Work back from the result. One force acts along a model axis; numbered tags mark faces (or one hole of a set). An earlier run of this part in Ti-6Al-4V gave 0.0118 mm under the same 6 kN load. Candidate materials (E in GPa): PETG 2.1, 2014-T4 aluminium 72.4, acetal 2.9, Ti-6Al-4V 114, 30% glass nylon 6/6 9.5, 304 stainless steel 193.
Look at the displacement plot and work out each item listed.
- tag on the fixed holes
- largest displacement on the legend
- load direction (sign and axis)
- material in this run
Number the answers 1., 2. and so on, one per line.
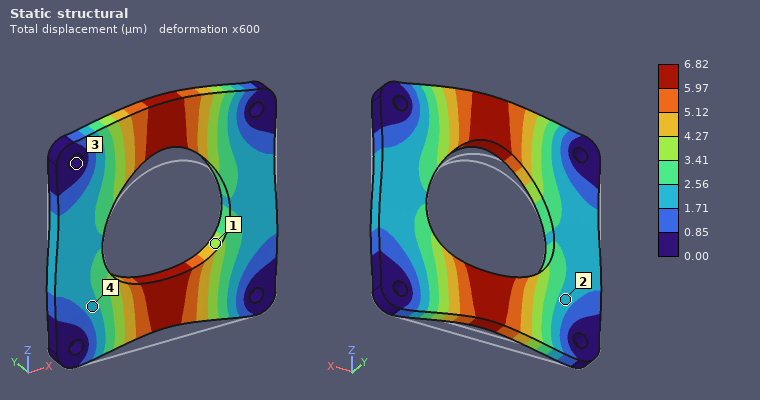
1. 3
2. 6.82 µm
3. +Z
4. 304 stainless steel
